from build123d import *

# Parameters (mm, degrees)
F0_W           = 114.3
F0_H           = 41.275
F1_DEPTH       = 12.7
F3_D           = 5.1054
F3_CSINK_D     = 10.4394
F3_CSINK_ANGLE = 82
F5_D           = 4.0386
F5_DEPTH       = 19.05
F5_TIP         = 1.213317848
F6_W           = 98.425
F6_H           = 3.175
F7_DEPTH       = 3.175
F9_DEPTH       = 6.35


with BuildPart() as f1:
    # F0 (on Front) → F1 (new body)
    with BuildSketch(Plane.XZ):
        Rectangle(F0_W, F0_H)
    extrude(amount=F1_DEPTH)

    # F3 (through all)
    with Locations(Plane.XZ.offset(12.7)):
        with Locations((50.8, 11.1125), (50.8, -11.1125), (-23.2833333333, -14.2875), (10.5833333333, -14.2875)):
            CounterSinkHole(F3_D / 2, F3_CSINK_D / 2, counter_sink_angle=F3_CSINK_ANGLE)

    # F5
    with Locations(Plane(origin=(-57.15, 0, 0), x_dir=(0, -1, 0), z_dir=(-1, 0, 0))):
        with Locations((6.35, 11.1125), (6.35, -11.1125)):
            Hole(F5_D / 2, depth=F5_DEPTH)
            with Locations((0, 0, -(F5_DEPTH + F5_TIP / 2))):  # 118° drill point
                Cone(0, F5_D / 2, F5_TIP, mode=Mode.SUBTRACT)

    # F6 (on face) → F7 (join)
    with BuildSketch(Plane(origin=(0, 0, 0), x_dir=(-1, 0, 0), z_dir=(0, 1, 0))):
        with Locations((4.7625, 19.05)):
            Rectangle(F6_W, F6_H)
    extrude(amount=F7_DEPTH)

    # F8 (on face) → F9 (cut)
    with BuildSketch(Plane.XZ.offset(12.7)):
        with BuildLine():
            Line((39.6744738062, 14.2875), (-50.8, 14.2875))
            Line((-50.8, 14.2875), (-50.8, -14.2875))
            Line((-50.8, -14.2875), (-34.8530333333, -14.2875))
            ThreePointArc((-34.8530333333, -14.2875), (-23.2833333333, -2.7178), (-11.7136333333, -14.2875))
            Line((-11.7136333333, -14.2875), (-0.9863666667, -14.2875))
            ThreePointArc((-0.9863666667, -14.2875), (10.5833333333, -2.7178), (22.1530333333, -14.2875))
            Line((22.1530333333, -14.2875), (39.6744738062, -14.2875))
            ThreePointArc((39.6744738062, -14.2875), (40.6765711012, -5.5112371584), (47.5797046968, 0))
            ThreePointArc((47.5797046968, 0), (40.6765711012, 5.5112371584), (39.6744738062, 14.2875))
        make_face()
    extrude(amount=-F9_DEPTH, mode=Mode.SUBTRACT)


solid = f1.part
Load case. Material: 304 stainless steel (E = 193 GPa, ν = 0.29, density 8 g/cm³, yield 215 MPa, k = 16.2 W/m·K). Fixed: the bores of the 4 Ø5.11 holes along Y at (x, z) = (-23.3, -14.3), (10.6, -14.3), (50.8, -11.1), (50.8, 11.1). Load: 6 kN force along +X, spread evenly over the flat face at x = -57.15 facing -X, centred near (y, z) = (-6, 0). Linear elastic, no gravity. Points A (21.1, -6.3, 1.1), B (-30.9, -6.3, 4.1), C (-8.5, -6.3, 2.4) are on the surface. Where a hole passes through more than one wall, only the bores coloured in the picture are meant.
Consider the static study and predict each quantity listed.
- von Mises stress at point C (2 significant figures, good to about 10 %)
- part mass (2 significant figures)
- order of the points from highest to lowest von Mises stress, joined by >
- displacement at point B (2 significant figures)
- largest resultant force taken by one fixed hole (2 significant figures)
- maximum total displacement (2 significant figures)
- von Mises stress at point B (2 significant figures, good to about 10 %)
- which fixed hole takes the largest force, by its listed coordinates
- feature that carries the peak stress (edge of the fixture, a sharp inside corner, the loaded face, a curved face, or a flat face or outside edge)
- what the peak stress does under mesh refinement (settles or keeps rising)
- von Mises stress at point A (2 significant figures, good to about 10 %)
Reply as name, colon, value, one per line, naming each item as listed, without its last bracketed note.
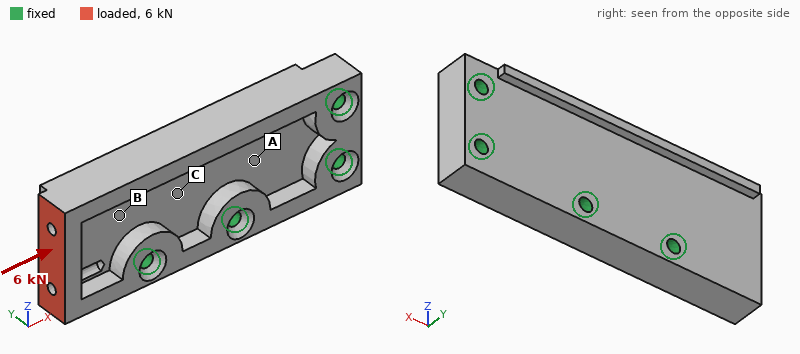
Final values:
von Mises stress at point C: 16 MPa
part mass: 360 g
order of the points from highest to lowest von Mises stress, joined by >: B > C > A
displacement at point B: 4.5 µm
largest resultant force taken by one fixed hole: 3.7 kN
maximum total displacement: 22 µm
von Mises stress at point B: 25 MPa
which fixed hole takes the largest force, by its listed coordinates: (-23.3, -14.3)
feature that carries the peak stress: edge of the fixture
what the peak stress does under mesh refinement: keeps rising
von Mises stress at point A: 6.1 MPa
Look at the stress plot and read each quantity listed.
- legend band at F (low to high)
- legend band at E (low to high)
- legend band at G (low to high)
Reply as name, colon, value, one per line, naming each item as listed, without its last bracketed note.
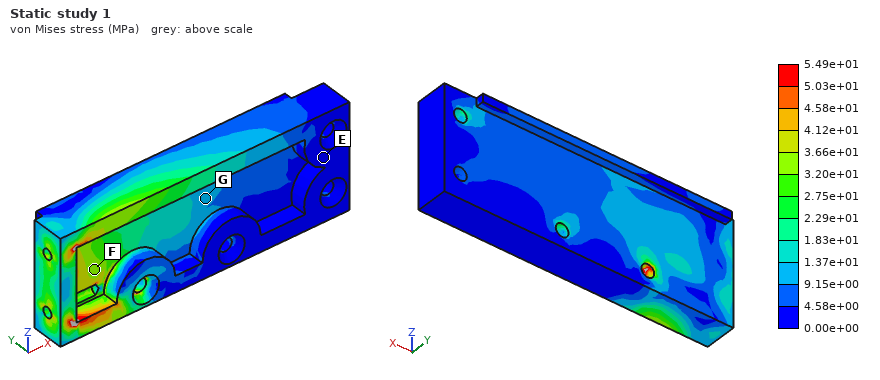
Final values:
legend band at F: 3.20e+01 to 3.66e+01 MPa
legend band at E: 0.00e+00 to 4.58e+00 MPa
legend band at G: 9.15e+00 to 1.37e+01 MPa
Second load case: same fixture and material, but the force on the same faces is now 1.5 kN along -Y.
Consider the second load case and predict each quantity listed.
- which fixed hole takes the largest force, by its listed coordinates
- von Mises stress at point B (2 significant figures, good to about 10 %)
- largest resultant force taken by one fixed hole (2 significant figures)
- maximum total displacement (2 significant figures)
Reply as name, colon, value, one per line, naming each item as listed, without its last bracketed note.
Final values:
which fixed hole takes the largest force, by its listed coordinates: (-23.3, -14.3)
von Mises stress at point B: 35 MPa
largest resultant force taken by one fixed hole: 2.0 kN
maximum total displacement: 80 µm
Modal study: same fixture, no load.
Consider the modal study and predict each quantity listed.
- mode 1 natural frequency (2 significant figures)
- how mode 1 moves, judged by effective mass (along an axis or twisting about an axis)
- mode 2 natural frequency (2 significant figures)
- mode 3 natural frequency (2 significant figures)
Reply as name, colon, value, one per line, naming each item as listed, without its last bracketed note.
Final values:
mode 1 natural frequency: 3300 Hz
how mode 1 moves, judged by effective mass: along Y
mode 2 natural frequency: 6200 Hz
mode 3 natural frequency: 8600 Hz
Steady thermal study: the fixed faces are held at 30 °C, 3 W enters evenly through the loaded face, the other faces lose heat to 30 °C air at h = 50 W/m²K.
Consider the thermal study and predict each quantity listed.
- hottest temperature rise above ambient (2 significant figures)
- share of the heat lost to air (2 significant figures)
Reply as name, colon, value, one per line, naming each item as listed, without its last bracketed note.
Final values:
hottest temperature rise above ambient: 14 K
share of the heat lost to air: 60 %
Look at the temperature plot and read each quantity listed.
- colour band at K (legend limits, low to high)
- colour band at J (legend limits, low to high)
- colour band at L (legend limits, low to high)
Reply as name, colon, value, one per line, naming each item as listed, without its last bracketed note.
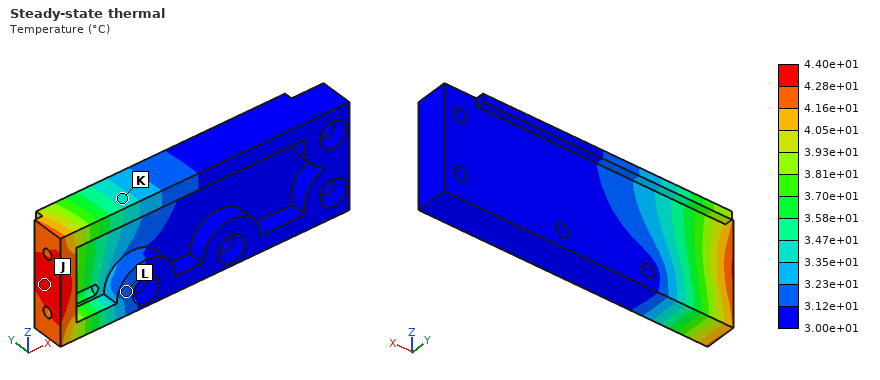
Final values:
colour band at K: 3.35e+01 to 3.47e+01 °C
colour band at J: 4.28e+01 to 4.40e+01 °C
colour band at L: 3.12e+01 to 3.23e+01 °C
